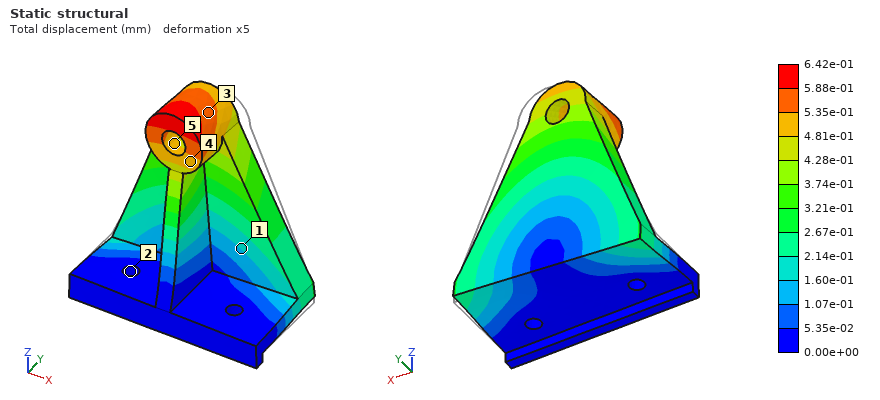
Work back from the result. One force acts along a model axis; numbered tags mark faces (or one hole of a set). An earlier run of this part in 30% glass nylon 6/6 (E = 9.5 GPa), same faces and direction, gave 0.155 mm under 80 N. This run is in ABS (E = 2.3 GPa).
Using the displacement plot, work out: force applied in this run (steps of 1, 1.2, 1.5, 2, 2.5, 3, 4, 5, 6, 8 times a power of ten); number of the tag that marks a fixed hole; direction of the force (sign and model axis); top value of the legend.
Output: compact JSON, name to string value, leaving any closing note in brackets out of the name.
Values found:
{"force applied in this run": "80 N", "number of the tag that marks a fixed hole": "2", "direction of the force": "-X", "top value of the legend": "6.42e-01 mm"}
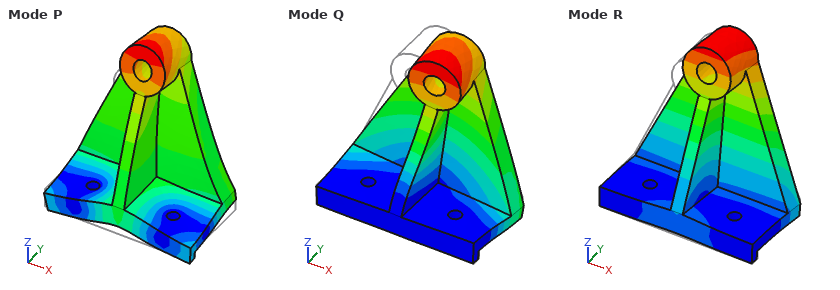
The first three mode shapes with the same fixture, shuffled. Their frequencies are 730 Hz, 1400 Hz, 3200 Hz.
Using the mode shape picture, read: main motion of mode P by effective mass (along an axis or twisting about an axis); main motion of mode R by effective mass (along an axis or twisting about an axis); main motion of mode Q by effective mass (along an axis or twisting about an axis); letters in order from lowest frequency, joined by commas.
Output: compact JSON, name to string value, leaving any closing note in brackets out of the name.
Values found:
{"main motion of mode P by effective mass": "along Z", "main motion of mode R by effective mass": "along Y", "main motion of mode Q by effective mass": "along X", "letters in order from lowest frequency, joined by commas": "R, Q, P"}
